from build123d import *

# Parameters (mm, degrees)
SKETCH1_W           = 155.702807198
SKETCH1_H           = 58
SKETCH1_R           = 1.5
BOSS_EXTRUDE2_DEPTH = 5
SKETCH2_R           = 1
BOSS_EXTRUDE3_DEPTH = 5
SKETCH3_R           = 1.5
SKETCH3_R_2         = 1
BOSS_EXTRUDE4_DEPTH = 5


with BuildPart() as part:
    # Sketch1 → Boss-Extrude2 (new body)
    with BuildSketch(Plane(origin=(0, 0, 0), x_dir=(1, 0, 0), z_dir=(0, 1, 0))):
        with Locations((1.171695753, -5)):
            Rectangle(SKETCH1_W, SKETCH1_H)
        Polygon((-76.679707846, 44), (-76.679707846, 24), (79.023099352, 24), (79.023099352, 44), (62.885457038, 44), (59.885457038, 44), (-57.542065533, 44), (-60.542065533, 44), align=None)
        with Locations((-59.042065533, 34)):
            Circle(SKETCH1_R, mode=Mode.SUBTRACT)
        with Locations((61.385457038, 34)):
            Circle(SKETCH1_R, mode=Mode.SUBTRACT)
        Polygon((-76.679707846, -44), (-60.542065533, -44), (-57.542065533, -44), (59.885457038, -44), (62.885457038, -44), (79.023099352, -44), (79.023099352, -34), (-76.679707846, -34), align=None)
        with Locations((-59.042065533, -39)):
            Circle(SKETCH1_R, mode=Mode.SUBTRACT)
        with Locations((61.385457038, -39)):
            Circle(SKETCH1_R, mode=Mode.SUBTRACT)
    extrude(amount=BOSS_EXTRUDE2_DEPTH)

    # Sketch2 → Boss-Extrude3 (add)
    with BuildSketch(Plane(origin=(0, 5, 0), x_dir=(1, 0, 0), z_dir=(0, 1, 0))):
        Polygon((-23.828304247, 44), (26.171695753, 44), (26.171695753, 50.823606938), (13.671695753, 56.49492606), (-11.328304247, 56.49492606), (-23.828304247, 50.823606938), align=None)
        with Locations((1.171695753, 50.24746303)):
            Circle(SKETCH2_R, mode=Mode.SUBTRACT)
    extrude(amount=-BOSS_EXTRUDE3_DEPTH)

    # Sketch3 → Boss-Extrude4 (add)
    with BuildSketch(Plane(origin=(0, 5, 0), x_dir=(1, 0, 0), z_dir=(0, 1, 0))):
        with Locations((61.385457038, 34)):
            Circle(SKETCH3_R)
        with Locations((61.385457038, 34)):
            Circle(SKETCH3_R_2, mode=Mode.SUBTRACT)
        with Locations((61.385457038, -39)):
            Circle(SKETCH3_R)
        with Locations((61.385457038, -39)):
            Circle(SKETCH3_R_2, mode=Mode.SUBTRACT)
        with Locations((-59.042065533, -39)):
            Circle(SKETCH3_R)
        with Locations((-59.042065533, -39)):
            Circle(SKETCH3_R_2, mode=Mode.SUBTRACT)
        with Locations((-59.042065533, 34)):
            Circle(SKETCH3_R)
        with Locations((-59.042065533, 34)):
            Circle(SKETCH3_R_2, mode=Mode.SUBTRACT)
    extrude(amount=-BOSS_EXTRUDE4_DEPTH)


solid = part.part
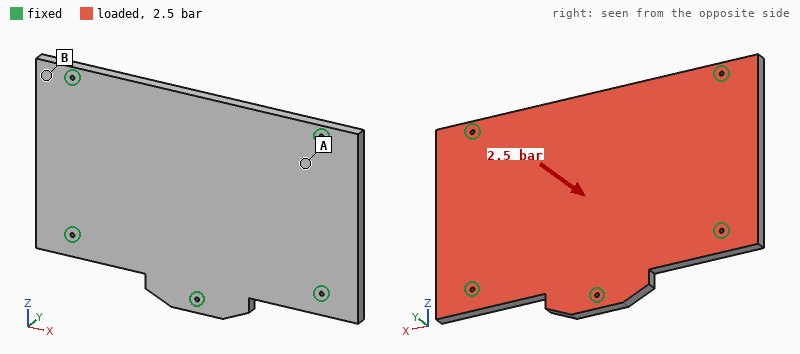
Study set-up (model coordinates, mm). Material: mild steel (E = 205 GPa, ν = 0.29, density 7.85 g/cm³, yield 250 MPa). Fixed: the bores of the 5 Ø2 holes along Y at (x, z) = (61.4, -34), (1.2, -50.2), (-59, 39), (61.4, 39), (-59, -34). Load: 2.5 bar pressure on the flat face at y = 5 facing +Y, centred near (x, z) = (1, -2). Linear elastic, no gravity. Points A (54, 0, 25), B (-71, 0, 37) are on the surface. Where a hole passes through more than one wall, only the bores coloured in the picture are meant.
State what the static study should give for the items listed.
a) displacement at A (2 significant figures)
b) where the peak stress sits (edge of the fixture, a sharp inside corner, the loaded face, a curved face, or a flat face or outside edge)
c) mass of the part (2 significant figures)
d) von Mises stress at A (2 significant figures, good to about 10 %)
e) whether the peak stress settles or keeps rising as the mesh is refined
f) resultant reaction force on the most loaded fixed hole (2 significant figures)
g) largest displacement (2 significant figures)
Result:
22 µm
edge of the fixture
560 g
31 MPa
keeps rising
810 N
99 µm
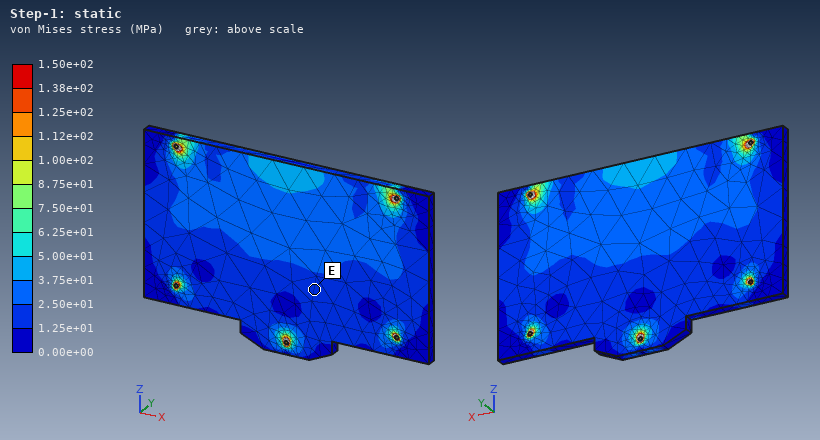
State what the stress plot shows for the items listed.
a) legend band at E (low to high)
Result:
1.25e+01 to 2.50e+01 MPa
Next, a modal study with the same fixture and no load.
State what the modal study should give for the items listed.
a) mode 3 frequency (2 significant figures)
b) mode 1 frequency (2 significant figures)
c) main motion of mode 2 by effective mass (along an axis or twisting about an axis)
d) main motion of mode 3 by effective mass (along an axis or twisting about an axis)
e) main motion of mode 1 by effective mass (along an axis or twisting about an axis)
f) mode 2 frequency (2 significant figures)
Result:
3500 Hz
1600 Hz
along Y
twisting about Z
along Y
3300 Hz
